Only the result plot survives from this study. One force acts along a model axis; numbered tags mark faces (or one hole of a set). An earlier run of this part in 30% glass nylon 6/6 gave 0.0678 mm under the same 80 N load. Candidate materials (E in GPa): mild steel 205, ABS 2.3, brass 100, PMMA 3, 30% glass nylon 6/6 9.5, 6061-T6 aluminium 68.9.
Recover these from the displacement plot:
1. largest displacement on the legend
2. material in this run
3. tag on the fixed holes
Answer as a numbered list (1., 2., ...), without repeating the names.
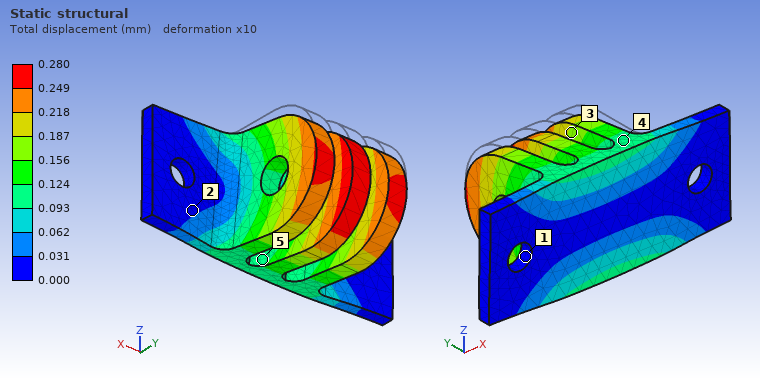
1. 0.280 mm
2. ABS
3. 1
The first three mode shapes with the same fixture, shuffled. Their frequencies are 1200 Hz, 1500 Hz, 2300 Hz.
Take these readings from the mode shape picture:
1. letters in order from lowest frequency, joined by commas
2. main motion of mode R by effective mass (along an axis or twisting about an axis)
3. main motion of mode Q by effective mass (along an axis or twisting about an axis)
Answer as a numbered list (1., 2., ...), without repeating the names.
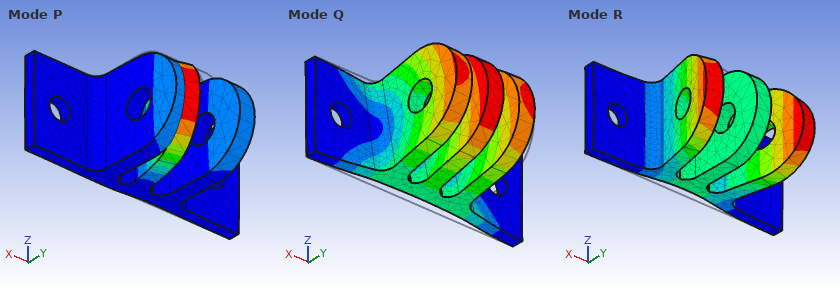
1. Q, R, P
2. along Y
3. along Z
